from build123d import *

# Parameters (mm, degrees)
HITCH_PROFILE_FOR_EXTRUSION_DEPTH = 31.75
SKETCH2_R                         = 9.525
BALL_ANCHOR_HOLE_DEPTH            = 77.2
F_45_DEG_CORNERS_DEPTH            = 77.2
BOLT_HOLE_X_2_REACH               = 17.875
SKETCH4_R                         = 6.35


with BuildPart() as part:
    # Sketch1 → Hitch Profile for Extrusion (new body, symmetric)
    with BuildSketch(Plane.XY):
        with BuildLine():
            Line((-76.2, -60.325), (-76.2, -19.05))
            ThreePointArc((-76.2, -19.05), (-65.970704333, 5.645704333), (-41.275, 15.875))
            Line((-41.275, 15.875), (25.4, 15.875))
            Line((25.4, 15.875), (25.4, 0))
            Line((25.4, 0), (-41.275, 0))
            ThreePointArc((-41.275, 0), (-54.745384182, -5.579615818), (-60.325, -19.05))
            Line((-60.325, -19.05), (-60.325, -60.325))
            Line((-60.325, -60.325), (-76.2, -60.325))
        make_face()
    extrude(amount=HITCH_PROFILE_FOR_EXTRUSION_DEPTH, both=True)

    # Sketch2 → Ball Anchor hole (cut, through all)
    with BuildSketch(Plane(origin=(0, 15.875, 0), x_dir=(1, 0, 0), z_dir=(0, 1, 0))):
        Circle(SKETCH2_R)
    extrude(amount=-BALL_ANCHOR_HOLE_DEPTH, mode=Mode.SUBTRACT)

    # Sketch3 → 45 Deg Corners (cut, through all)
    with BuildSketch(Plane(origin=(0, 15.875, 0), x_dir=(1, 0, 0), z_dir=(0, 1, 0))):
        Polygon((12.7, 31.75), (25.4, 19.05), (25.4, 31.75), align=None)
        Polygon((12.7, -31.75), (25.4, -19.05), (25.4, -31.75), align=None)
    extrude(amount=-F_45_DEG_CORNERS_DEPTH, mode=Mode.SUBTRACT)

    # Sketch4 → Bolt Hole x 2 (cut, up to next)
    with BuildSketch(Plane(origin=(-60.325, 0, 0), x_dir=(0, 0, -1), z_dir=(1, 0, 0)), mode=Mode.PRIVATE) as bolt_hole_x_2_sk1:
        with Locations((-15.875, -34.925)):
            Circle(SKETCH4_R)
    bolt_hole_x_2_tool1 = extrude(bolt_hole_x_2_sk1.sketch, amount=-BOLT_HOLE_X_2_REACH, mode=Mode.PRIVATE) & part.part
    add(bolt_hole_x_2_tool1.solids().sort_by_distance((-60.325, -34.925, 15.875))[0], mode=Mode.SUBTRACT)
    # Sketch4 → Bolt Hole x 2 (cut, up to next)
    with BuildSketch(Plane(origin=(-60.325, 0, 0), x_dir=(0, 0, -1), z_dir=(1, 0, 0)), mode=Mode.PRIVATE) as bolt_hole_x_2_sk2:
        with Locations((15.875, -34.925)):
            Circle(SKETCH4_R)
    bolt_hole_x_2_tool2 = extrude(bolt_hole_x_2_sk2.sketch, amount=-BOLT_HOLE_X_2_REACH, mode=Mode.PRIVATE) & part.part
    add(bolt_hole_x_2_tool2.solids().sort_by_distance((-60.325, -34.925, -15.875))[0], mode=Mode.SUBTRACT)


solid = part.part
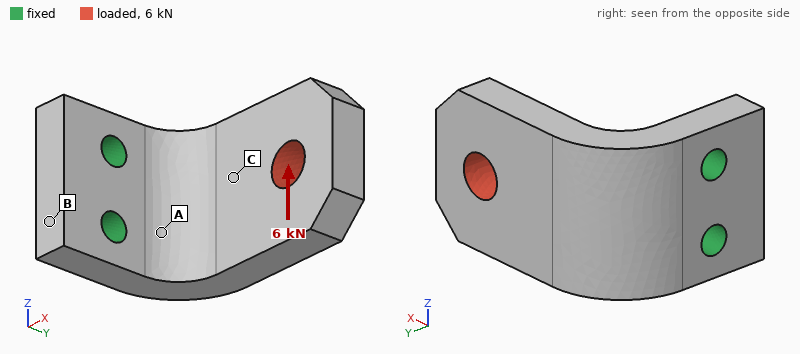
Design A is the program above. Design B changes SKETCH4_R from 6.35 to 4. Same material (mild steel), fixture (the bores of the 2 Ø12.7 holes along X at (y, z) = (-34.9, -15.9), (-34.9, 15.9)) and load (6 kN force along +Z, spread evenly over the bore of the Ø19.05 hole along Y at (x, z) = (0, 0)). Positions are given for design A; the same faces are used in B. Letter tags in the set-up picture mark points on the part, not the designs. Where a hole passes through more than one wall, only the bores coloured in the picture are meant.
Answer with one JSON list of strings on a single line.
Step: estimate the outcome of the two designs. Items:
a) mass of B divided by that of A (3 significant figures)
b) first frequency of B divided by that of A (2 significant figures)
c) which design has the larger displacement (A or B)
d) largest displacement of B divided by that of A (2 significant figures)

["1.02", "0.95", "B", "1.1"]
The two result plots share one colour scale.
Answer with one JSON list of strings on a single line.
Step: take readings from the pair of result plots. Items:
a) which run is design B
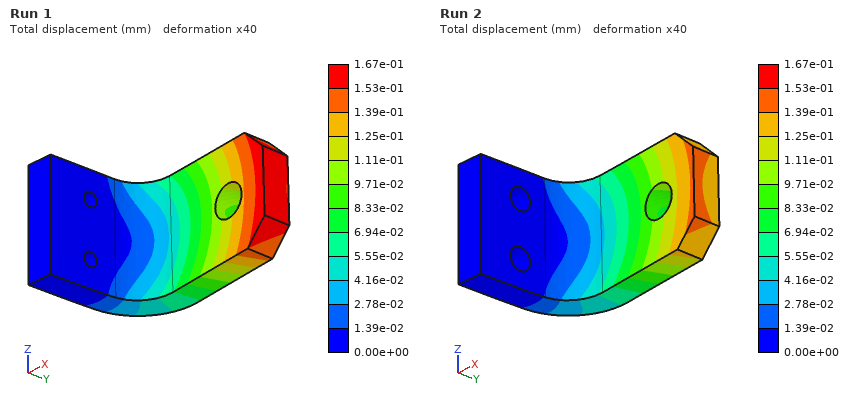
["Run 1"]
